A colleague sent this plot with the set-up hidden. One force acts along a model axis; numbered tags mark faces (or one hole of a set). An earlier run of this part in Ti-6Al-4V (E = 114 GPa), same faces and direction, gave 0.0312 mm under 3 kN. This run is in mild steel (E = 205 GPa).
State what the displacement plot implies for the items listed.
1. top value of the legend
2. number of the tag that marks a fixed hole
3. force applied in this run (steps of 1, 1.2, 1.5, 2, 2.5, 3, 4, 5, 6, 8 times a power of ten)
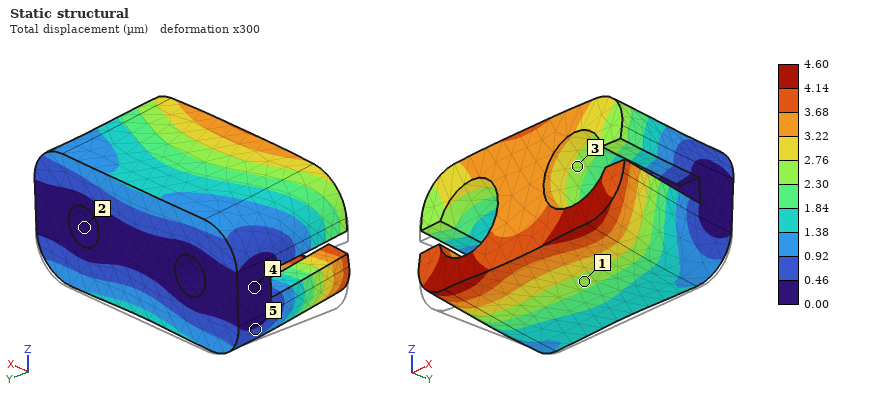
4.60 µm
2
800 N
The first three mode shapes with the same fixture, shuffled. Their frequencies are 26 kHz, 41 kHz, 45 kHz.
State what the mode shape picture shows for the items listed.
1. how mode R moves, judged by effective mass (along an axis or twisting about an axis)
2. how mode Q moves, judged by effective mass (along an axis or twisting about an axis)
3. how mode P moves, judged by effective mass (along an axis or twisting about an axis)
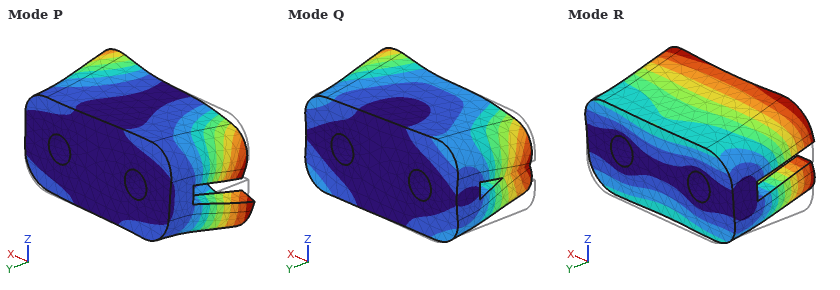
along Z
along X
twisting about Y
